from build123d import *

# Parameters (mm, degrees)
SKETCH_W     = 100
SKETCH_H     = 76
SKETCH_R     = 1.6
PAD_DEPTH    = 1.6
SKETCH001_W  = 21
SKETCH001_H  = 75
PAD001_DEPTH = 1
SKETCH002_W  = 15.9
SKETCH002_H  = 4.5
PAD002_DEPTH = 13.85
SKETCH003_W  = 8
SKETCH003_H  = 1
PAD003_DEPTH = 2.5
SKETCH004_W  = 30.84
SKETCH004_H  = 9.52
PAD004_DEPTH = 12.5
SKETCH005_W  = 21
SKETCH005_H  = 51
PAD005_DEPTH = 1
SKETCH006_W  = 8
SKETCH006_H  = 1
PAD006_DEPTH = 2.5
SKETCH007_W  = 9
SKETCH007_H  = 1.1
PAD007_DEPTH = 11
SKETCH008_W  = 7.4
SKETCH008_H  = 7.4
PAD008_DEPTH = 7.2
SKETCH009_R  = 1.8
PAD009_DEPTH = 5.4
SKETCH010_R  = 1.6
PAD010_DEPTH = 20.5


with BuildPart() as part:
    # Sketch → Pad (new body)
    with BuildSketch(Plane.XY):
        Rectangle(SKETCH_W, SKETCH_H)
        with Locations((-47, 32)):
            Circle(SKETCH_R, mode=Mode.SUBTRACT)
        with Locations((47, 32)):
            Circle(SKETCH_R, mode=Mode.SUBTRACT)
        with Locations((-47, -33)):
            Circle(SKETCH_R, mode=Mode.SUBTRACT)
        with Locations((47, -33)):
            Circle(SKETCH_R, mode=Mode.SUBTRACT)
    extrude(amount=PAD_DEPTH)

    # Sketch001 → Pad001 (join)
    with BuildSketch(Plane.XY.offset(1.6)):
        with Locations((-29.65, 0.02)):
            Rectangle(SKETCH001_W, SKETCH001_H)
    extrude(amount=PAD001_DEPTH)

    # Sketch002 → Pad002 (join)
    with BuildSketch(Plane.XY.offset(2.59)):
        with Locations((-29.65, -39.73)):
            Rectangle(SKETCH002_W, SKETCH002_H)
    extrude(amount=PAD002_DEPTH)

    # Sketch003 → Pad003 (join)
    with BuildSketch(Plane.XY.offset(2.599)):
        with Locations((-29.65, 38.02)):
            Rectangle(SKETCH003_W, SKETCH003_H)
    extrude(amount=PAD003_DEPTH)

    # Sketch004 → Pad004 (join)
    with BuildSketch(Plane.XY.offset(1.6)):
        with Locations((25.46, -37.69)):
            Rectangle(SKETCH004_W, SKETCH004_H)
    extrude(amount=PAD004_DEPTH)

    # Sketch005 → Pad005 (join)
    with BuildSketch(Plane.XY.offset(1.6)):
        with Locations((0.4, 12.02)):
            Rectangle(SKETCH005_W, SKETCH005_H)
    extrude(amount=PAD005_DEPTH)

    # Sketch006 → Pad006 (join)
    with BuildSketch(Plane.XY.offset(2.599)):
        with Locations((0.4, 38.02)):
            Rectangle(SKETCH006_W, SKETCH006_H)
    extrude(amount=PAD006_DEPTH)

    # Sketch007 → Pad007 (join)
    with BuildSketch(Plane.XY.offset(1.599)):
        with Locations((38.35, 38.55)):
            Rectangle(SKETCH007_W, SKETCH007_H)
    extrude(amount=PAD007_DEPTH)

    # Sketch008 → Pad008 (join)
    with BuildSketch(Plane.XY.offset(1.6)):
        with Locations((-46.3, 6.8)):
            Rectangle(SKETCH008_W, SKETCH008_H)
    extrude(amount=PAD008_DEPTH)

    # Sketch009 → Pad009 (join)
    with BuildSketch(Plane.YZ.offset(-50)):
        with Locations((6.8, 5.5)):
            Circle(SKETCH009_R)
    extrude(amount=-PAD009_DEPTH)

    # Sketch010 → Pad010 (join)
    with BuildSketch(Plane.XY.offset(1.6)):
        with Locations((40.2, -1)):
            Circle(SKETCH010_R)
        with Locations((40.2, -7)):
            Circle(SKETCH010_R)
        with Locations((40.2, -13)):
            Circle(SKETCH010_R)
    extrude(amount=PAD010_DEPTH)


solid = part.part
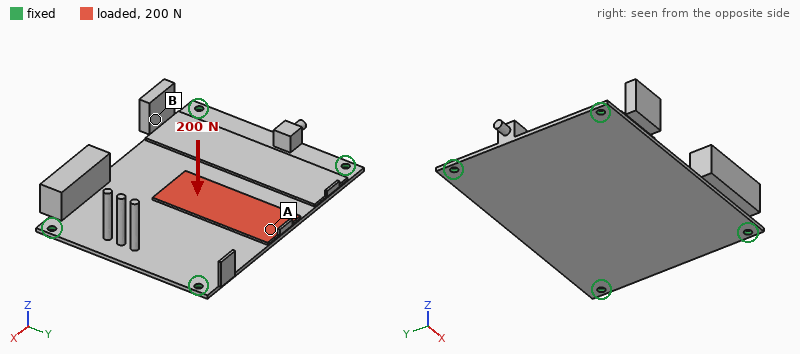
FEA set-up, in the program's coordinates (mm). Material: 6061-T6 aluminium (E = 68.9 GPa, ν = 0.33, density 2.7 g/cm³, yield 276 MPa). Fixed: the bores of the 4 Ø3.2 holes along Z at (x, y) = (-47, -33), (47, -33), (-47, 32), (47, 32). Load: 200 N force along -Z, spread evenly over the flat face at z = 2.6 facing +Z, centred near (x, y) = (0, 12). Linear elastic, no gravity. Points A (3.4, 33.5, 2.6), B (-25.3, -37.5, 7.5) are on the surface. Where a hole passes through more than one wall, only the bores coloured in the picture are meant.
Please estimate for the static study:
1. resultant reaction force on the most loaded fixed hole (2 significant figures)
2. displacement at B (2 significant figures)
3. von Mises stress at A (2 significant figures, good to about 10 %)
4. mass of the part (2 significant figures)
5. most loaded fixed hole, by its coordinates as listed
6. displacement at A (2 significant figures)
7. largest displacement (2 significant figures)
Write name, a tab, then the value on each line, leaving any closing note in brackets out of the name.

resultant reaction force on the most loaded fixed hole	160 N
displacement at B	0.17 mm
von Mises stress at A	40 MPa
mass of the part	55 g
most loaded fixed hole, by its coordinates as listed	(-47, 32)
displacement at A	0.49 mm
largest displacement	0.51 mm
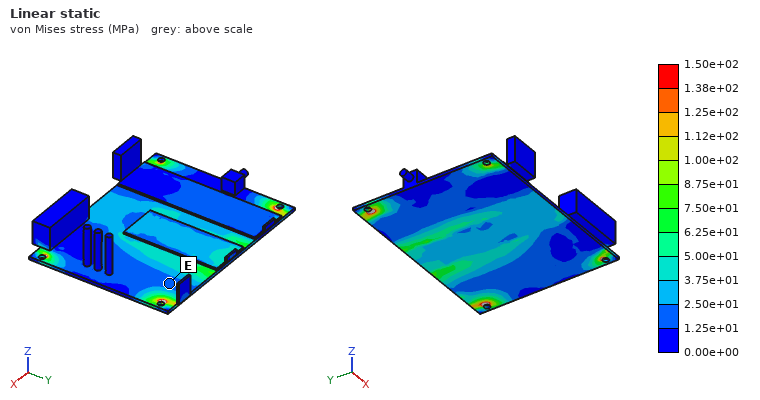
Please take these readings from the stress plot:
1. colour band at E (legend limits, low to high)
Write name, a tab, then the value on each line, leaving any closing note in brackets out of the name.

colour band at E	1.25e+01 to 2.50e+01 MPa
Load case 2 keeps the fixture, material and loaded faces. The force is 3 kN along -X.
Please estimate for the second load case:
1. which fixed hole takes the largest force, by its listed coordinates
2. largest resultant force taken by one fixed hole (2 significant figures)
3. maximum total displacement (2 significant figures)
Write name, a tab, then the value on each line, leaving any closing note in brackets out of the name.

which fixed hole takes the largest force, by its listed coordinates	(-47, 32)
largest resultant force taken by one fixed hole	1000 N
maximum total displacement	0.15 mm
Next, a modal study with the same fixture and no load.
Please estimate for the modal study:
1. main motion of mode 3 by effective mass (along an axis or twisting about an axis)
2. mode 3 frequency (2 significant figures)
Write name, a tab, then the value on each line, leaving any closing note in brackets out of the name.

main motion of mode 3 by effective mass	along Z
mode 3 frequency	690 Hz
